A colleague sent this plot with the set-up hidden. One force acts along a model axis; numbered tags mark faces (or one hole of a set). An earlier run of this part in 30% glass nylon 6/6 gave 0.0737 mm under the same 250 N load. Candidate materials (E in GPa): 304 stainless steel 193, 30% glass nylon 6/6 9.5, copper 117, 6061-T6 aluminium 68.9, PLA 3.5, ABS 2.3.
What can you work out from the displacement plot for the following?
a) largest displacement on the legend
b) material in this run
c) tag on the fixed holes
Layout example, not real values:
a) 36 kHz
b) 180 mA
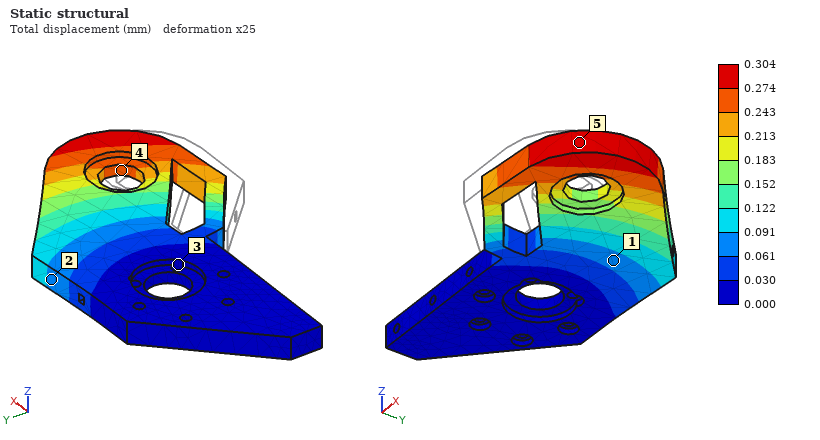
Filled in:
a) 0.304 mm
b) ABS
c) 3
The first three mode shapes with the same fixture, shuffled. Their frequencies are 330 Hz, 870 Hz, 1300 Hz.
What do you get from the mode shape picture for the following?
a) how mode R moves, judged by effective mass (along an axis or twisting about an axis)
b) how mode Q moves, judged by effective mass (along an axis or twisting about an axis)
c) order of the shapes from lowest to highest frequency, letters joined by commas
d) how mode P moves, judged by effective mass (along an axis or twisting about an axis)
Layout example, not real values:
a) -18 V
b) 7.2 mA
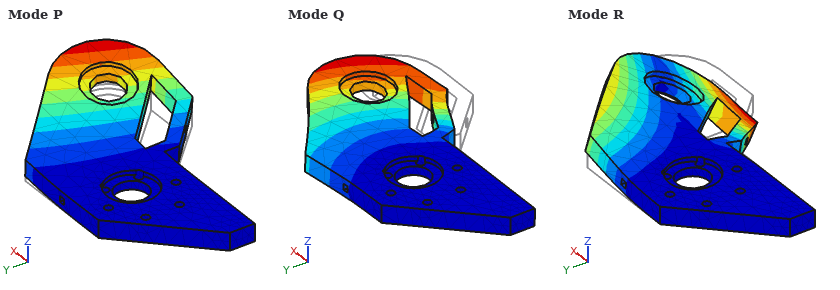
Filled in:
a) twisting about X
b) along Y
c) P, R, Q
d) along Z
